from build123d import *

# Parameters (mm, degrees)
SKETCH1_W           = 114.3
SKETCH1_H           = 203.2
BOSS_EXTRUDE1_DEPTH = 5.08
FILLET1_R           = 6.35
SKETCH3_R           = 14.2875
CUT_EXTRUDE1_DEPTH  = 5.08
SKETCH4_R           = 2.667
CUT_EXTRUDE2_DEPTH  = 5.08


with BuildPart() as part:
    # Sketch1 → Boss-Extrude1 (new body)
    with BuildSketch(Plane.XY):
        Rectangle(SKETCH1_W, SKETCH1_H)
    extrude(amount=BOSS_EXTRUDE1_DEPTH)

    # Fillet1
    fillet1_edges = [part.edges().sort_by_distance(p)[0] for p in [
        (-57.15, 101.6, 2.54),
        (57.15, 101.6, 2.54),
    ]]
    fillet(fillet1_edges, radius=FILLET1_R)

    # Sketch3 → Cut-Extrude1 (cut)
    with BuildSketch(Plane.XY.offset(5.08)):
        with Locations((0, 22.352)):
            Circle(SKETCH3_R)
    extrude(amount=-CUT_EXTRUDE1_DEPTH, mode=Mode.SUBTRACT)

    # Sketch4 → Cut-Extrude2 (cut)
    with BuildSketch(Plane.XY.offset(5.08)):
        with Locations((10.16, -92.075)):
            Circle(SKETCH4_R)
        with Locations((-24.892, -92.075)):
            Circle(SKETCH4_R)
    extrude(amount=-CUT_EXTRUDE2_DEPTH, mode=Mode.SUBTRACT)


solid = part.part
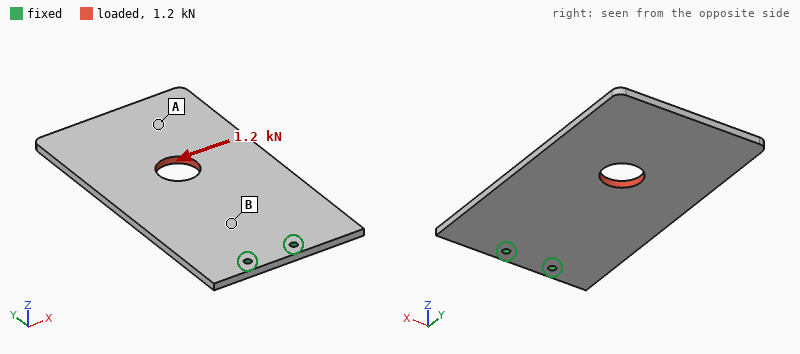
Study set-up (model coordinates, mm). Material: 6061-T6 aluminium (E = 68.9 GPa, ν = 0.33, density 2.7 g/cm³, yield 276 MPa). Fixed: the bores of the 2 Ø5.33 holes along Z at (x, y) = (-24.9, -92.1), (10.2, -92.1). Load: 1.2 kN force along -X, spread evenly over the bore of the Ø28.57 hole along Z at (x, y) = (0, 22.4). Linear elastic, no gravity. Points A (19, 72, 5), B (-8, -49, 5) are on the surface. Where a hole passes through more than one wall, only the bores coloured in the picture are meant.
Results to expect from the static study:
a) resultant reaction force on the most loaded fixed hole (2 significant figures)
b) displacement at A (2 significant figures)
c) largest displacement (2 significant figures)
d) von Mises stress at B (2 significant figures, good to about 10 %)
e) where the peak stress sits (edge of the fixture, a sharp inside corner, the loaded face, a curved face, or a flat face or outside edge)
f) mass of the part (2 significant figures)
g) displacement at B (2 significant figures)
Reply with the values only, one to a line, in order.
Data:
3.6 kN
0.13 mm
0.16 mm
10 MPa
edge of the fixture
310 g
0.032 mm
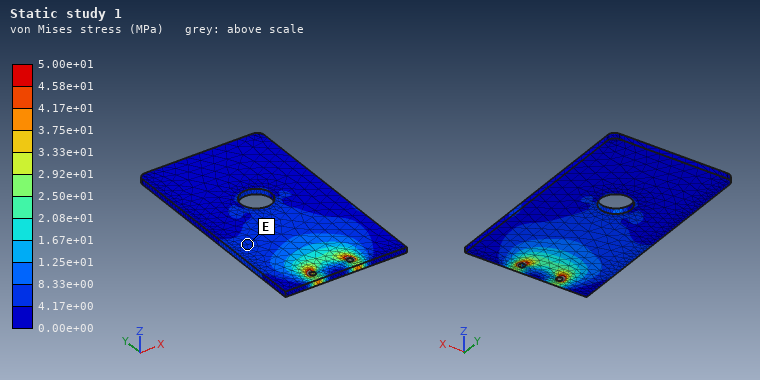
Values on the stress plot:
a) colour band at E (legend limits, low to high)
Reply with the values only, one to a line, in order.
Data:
4.17e+00 to 8.33e+00 MPa
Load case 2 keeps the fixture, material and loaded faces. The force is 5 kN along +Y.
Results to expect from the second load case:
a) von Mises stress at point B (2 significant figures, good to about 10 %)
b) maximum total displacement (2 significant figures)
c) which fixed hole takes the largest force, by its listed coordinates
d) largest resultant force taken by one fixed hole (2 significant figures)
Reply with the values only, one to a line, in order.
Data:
13 MPa
48 µm
(10.2, -92.1)
3.5 kN
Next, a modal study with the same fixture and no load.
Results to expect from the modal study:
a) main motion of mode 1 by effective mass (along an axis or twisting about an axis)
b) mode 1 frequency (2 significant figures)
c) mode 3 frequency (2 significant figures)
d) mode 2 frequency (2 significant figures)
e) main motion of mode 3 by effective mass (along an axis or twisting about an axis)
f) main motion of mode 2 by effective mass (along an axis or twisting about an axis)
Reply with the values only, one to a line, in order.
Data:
along Z
110 Hz
630 Hz
360 Hz
along Z
twisting about Y
